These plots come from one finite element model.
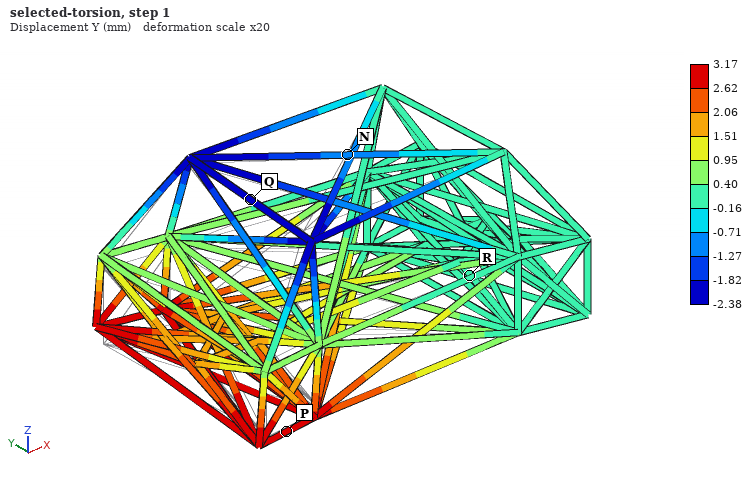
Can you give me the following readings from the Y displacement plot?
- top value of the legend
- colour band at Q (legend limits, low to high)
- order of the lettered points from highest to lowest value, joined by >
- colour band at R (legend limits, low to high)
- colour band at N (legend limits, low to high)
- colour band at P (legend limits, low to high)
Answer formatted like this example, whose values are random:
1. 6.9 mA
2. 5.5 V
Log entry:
1. 3.17 mm
2. -2.38 to -1.82 mm
3. P > R > N > Q
4. -0.16 to 0.40 mm
5. -1.27 to -0.71 mm
6. 2.62 to 3.17 mm
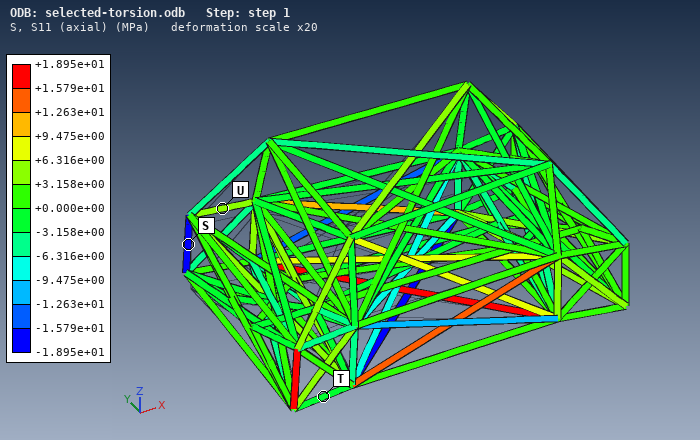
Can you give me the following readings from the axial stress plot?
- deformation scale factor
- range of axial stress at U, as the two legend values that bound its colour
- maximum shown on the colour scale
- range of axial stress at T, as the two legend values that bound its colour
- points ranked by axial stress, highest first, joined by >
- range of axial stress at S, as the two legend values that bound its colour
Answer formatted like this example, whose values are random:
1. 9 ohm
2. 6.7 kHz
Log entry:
1. 20
2. +3.158e+00 to +6.316e+00 MPa
3. +1.895e+01 MPa
4. -3.158e+00 to +0.000e+00 MPa
5. U > T > S
6. -1.895e+01 to -1.579e+01 MPa
